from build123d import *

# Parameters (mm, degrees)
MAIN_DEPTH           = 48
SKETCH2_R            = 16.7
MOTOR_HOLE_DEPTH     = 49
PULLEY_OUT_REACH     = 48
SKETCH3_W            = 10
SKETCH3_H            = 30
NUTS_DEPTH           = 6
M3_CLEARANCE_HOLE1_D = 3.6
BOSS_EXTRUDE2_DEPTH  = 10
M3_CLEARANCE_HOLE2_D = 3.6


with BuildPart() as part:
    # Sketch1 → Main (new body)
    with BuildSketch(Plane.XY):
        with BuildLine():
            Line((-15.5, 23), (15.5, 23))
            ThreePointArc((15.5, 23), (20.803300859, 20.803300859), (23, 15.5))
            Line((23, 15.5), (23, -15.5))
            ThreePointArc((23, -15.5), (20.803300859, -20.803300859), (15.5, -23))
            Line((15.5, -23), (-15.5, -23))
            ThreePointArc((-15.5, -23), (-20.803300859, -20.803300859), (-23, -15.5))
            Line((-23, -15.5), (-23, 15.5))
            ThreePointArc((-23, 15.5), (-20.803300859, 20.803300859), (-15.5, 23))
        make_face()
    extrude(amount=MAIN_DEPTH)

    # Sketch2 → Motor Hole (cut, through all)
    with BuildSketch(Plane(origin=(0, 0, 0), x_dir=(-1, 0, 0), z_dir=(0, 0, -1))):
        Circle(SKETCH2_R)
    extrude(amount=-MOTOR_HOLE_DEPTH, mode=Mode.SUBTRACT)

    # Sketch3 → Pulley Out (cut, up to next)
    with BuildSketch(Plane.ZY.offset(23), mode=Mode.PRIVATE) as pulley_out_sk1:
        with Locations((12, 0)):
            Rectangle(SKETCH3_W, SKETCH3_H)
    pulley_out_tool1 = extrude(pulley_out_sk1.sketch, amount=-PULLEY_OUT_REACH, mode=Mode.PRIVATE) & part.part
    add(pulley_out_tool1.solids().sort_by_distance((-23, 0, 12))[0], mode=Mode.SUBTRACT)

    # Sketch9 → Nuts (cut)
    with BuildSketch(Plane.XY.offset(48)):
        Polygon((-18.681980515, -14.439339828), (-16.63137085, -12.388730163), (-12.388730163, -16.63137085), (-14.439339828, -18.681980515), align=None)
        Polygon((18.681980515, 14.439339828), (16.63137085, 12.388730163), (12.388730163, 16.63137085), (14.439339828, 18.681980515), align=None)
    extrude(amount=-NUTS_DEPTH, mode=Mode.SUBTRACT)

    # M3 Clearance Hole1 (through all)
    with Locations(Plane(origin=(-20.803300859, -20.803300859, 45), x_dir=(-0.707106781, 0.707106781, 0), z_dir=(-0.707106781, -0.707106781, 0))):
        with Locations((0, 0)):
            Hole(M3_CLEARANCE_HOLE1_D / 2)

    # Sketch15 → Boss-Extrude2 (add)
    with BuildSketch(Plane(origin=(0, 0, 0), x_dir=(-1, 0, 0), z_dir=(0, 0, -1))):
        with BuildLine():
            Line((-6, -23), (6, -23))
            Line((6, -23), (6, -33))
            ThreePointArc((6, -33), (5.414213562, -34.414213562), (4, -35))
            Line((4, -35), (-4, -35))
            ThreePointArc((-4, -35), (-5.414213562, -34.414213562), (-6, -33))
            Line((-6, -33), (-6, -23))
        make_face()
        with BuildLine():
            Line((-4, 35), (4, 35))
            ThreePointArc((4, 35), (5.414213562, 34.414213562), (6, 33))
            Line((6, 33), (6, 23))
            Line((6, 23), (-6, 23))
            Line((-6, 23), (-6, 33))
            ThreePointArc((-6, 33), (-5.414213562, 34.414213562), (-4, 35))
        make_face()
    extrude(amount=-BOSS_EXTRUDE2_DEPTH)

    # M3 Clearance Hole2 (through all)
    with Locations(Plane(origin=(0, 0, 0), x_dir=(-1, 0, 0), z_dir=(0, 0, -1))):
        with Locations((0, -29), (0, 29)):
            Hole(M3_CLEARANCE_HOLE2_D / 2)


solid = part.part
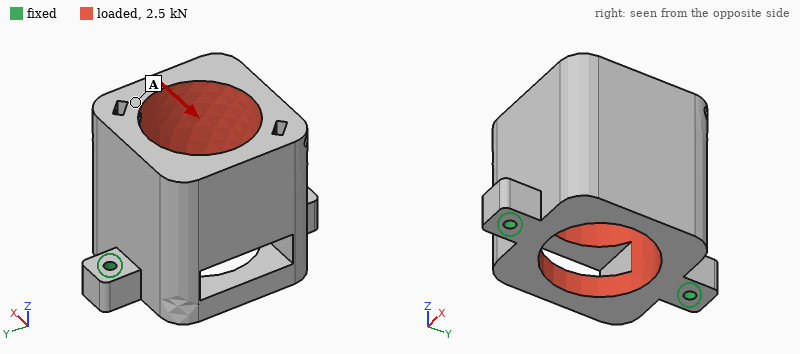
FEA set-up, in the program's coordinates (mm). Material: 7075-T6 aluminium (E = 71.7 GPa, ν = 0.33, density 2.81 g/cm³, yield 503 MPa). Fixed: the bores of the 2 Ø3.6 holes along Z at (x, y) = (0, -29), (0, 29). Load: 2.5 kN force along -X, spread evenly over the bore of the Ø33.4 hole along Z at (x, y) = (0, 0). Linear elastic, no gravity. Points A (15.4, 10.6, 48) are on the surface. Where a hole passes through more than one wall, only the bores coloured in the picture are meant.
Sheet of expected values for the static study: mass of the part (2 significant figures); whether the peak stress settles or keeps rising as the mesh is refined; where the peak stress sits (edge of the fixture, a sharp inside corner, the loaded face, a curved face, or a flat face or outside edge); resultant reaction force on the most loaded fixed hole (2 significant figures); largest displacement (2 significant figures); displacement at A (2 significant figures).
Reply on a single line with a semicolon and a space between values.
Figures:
160 g; keeps rising; edge of the fixture; 1.3 kN; 0.19 mm; 0.18 mm
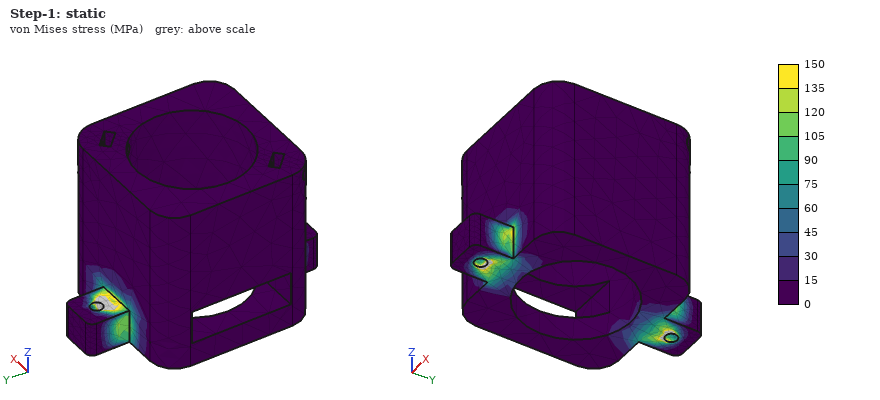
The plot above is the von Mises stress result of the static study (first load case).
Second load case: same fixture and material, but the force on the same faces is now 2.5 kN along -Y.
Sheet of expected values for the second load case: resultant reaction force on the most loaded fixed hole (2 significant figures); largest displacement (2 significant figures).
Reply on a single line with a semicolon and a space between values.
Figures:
1.6 kN; 15 µm
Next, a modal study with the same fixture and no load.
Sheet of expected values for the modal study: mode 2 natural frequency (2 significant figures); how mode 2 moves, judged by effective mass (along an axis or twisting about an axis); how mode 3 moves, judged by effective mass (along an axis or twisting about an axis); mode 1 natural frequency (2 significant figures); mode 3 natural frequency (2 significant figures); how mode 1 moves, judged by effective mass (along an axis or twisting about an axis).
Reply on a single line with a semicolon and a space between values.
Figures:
6000 Hz; along Y; along Z; 1600 Hz; 7500 Hz; along X
